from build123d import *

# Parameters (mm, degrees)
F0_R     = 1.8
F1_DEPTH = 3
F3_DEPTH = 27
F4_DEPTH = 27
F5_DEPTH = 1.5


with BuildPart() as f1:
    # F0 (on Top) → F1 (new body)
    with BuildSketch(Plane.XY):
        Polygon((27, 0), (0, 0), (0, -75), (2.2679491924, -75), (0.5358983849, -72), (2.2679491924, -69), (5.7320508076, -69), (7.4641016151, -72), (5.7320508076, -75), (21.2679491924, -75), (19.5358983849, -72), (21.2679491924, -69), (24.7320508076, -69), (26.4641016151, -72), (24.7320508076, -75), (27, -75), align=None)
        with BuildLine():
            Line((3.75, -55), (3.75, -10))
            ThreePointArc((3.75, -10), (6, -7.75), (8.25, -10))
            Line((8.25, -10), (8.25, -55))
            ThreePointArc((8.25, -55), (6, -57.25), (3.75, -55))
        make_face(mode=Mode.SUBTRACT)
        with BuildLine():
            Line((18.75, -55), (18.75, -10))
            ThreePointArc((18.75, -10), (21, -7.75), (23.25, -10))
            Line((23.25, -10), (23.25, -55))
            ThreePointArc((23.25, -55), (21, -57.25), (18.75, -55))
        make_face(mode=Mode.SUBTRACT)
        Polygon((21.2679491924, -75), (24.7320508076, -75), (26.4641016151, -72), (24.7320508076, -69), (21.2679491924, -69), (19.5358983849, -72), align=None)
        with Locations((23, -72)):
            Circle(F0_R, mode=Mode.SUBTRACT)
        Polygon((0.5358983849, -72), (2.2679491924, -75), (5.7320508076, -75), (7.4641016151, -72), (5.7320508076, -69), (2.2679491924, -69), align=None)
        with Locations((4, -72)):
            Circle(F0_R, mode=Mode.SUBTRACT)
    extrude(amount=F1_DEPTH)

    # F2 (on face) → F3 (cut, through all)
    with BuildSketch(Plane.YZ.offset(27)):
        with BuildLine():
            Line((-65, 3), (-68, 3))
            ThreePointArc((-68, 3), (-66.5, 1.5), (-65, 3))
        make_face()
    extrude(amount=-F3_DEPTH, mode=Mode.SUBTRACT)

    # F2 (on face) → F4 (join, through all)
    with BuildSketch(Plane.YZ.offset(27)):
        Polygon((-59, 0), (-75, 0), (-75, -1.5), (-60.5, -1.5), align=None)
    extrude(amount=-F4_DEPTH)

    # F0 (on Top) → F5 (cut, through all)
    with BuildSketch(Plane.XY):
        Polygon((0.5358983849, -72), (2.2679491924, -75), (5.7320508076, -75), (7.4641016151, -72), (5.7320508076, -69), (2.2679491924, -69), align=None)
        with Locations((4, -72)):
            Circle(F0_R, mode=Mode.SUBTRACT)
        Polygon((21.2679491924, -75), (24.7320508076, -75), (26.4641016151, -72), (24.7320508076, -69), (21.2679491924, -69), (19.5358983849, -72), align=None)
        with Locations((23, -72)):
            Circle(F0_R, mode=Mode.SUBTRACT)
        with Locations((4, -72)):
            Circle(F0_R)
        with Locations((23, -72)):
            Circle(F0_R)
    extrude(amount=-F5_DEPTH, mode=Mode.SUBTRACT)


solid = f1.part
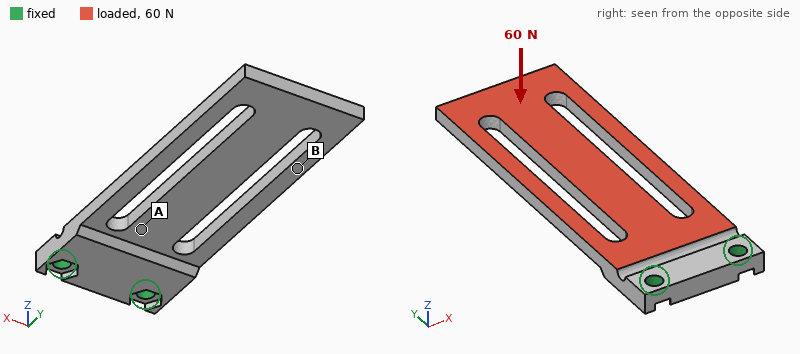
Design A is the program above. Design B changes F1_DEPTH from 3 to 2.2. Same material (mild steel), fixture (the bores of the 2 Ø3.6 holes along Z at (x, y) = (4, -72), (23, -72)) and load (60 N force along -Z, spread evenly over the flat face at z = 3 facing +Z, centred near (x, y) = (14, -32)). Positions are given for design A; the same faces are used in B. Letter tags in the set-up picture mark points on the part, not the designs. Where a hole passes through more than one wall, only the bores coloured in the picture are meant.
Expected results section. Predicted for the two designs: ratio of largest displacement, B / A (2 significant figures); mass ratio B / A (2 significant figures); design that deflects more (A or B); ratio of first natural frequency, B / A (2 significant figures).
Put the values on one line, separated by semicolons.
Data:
2.2; 0.77; B; 0.79
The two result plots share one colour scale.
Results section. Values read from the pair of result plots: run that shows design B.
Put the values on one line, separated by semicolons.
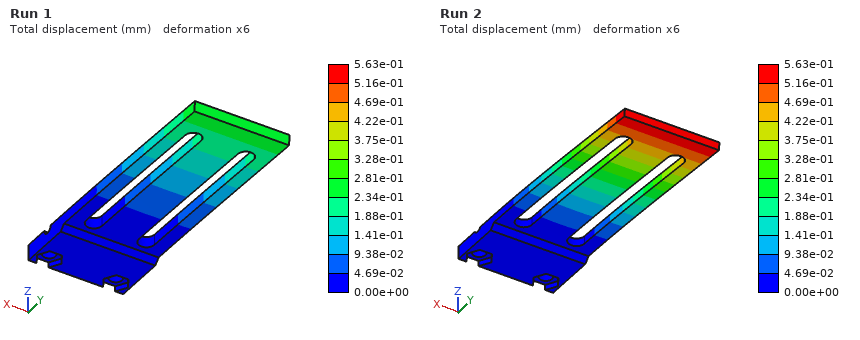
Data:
Run 2
